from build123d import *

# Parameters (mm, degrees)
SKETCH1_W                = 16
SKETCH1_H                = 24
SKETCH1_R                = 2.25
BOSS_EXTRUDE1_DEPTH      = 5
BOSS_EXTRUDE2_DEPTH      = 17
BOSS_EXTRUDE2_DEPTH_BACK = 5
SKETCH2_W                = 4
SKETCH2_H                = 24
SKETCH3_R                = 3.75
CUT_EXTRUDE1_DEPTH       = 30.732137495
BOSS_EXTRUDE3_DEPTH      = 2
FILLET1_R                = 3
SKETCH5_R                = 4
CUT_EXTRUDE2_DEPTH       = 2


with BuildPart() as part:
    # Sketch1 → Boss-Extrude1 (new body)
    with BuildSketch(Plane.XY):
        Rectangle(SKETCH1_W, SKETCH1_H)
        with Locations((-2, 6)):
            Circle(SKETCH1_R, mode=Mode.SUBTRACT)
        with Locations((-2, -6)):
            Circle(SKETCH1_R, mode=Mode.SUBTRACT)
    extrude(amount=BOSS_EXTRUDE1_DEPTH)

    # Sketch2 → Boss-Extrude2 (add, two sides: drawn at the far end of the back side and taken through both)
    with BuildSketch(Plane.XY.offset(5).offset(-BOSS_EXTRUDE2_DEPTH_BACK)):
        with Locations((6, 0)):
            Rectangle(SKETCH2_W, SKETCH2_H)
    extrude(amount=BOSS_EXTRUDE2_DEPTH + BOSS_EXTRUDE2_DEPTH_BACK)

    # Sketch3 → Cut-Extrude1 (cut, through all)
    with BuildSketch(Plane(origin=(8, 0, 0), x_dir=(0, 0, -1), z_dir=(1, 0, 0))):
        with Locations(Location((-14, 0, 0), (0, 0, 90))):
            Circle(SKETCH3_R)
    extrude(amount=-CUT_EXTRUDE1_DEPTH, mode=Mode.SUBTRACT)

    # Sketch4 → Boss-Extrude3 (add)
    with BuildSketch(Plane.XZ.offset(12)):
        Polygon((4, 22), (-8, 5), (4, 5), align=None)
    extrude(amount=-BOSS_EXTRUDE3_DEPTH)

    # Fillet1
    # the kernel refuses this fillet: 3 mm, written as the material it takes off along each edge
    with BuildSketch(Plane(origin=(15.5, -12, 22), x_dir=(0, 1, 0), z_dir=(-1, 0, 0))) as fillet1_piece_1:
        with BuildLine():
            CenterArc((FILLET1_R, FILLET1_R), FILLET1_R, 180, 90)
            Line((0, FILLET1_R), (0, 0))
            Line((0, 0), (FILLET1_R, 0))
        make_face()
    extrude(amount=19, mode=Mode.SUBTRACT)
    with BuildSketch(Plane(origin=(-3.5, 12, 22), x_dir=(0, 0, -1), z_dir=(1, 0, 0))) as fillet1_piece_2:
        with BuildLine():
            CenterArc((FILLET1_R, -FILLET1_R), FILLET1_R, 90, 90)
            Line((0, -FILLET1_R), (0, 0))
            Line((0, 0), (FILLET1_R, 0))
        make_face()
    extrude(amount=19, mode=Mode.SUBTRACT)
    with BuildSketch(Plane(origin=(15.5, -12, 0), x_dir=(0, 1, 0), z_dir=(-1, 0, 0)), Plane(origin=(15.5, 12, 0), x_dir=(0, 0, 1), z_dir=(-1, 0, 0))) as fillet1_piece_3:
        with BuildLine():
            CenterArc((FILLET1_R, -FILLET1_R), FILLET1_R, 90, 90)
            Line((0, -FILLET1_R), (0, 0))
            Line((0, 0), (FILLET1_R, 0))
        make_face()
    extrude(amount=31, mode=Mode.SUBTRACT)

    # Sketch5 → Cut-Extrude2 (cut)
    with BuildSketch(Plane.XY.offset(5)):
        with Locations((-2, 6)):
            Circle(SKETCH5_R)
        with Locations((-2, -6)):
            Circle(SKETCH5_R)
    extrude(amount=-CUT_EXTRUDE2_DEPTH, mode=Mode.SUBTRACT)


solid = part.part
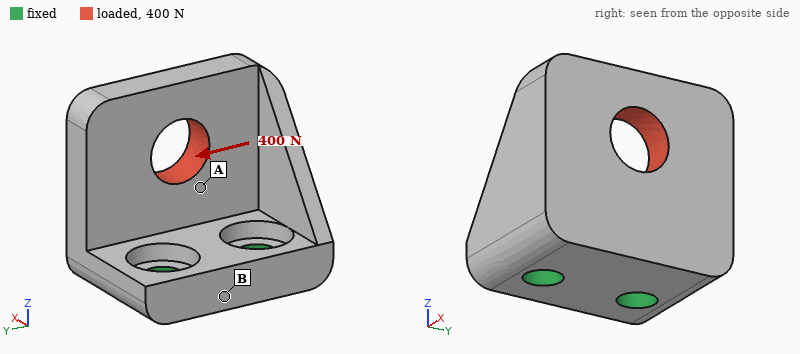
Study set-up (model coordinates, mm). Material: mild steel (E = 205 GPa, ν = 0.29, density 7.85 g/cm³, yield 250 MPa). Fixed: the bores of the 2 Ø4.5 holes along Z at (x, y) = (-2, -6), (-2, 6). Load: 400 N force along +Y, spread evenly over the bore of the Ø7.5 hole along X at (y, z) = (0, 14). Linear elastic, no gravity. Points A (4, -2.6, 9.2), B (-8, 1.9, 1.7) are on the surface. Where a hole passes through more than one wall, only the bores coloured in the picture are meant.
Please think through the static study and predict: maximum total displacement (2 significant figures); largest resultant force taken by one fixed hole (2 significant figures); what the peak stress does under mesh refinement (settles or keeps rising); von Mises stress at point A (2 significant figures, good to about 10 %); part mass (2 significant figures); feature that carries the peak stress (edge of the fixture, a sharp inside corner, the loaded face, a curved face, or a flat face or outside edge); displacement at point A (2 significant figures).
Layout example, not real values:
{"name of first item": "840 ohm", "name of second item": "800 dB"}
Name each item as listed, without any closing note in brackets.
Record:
{"maximum total displacement": "8.1 µm", "largest resultant force taken by one fixed hole": "440 N", "what the peak stress does under mesh refinement": "keeps rising", "von Mises stress at point A": "20 MPa", "part mass": "25 g", "feature that carries the peak stress": "edge of the fixture", "displacement at point A": "2.7 µm"}
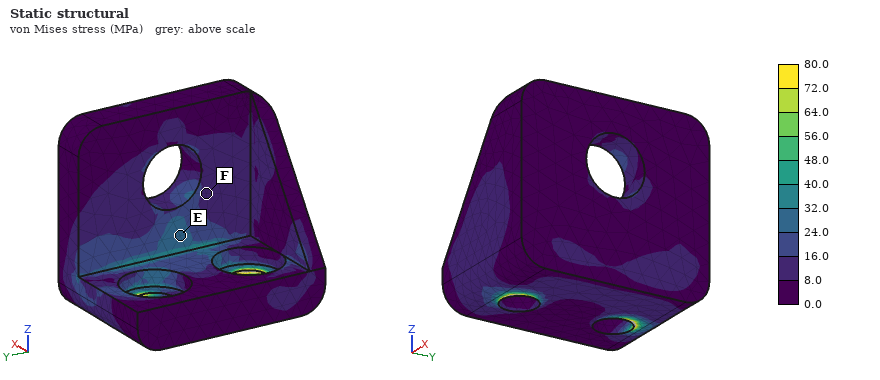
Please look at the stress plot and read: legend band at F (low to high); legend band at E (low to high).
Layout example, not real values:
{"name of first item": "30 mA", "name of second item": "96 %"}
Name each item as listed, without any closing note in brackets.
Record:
{"legend band at F": "8.0 to 16.0 MPa", "legend band at E": "24.0 to 32.0 MPa"}
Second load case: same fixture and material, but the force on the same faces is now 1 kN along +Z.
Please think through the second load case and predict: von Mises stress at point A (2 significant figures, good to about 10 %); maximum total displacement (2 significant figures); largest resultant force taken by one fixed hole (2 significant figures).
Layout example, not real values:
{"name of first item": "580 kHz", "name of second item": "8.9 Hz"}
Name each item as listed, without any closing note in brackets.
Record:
{"von Mises stress at point A": "22 MPa", "maximum total displacement": "21 µm", "largest resultant force taken by one fixed hole": "500 N"}
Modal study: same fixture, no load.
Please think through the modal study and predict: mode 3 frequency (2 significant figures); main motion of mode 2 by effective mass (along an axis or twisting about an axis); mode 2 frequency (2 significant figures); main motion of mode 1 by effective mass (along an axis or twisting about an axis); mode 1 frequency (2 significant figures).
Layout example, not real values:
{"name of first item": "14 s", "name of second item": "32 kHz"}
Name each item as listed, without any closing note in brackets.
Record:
{"mode 3 frequency": "18 kHz", "main motion of mode 2 by effective mass": "along Y", "mode 2 frequency": "11 kHz", "main motion of mode 1 by effective mass": "along X", "mode 1 frequency": "7100 Hz"}
